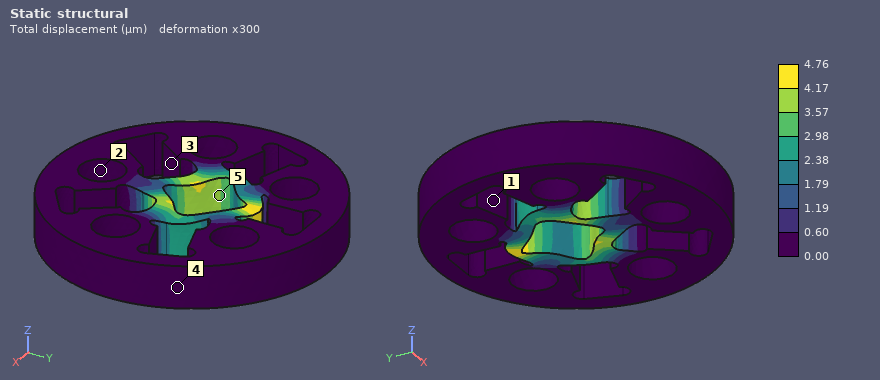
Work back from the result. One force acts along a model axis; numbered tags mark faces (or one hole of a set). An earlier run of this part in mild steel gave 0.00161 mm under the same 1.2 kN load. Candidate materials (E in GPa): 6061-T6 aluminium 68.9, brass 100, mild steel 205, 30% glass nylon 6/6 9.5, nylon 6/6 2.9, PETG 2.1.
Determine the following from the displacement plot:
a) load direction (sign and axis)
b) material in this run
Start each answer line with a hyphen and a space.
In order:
- +Y
- 6061-T6 aluminium
